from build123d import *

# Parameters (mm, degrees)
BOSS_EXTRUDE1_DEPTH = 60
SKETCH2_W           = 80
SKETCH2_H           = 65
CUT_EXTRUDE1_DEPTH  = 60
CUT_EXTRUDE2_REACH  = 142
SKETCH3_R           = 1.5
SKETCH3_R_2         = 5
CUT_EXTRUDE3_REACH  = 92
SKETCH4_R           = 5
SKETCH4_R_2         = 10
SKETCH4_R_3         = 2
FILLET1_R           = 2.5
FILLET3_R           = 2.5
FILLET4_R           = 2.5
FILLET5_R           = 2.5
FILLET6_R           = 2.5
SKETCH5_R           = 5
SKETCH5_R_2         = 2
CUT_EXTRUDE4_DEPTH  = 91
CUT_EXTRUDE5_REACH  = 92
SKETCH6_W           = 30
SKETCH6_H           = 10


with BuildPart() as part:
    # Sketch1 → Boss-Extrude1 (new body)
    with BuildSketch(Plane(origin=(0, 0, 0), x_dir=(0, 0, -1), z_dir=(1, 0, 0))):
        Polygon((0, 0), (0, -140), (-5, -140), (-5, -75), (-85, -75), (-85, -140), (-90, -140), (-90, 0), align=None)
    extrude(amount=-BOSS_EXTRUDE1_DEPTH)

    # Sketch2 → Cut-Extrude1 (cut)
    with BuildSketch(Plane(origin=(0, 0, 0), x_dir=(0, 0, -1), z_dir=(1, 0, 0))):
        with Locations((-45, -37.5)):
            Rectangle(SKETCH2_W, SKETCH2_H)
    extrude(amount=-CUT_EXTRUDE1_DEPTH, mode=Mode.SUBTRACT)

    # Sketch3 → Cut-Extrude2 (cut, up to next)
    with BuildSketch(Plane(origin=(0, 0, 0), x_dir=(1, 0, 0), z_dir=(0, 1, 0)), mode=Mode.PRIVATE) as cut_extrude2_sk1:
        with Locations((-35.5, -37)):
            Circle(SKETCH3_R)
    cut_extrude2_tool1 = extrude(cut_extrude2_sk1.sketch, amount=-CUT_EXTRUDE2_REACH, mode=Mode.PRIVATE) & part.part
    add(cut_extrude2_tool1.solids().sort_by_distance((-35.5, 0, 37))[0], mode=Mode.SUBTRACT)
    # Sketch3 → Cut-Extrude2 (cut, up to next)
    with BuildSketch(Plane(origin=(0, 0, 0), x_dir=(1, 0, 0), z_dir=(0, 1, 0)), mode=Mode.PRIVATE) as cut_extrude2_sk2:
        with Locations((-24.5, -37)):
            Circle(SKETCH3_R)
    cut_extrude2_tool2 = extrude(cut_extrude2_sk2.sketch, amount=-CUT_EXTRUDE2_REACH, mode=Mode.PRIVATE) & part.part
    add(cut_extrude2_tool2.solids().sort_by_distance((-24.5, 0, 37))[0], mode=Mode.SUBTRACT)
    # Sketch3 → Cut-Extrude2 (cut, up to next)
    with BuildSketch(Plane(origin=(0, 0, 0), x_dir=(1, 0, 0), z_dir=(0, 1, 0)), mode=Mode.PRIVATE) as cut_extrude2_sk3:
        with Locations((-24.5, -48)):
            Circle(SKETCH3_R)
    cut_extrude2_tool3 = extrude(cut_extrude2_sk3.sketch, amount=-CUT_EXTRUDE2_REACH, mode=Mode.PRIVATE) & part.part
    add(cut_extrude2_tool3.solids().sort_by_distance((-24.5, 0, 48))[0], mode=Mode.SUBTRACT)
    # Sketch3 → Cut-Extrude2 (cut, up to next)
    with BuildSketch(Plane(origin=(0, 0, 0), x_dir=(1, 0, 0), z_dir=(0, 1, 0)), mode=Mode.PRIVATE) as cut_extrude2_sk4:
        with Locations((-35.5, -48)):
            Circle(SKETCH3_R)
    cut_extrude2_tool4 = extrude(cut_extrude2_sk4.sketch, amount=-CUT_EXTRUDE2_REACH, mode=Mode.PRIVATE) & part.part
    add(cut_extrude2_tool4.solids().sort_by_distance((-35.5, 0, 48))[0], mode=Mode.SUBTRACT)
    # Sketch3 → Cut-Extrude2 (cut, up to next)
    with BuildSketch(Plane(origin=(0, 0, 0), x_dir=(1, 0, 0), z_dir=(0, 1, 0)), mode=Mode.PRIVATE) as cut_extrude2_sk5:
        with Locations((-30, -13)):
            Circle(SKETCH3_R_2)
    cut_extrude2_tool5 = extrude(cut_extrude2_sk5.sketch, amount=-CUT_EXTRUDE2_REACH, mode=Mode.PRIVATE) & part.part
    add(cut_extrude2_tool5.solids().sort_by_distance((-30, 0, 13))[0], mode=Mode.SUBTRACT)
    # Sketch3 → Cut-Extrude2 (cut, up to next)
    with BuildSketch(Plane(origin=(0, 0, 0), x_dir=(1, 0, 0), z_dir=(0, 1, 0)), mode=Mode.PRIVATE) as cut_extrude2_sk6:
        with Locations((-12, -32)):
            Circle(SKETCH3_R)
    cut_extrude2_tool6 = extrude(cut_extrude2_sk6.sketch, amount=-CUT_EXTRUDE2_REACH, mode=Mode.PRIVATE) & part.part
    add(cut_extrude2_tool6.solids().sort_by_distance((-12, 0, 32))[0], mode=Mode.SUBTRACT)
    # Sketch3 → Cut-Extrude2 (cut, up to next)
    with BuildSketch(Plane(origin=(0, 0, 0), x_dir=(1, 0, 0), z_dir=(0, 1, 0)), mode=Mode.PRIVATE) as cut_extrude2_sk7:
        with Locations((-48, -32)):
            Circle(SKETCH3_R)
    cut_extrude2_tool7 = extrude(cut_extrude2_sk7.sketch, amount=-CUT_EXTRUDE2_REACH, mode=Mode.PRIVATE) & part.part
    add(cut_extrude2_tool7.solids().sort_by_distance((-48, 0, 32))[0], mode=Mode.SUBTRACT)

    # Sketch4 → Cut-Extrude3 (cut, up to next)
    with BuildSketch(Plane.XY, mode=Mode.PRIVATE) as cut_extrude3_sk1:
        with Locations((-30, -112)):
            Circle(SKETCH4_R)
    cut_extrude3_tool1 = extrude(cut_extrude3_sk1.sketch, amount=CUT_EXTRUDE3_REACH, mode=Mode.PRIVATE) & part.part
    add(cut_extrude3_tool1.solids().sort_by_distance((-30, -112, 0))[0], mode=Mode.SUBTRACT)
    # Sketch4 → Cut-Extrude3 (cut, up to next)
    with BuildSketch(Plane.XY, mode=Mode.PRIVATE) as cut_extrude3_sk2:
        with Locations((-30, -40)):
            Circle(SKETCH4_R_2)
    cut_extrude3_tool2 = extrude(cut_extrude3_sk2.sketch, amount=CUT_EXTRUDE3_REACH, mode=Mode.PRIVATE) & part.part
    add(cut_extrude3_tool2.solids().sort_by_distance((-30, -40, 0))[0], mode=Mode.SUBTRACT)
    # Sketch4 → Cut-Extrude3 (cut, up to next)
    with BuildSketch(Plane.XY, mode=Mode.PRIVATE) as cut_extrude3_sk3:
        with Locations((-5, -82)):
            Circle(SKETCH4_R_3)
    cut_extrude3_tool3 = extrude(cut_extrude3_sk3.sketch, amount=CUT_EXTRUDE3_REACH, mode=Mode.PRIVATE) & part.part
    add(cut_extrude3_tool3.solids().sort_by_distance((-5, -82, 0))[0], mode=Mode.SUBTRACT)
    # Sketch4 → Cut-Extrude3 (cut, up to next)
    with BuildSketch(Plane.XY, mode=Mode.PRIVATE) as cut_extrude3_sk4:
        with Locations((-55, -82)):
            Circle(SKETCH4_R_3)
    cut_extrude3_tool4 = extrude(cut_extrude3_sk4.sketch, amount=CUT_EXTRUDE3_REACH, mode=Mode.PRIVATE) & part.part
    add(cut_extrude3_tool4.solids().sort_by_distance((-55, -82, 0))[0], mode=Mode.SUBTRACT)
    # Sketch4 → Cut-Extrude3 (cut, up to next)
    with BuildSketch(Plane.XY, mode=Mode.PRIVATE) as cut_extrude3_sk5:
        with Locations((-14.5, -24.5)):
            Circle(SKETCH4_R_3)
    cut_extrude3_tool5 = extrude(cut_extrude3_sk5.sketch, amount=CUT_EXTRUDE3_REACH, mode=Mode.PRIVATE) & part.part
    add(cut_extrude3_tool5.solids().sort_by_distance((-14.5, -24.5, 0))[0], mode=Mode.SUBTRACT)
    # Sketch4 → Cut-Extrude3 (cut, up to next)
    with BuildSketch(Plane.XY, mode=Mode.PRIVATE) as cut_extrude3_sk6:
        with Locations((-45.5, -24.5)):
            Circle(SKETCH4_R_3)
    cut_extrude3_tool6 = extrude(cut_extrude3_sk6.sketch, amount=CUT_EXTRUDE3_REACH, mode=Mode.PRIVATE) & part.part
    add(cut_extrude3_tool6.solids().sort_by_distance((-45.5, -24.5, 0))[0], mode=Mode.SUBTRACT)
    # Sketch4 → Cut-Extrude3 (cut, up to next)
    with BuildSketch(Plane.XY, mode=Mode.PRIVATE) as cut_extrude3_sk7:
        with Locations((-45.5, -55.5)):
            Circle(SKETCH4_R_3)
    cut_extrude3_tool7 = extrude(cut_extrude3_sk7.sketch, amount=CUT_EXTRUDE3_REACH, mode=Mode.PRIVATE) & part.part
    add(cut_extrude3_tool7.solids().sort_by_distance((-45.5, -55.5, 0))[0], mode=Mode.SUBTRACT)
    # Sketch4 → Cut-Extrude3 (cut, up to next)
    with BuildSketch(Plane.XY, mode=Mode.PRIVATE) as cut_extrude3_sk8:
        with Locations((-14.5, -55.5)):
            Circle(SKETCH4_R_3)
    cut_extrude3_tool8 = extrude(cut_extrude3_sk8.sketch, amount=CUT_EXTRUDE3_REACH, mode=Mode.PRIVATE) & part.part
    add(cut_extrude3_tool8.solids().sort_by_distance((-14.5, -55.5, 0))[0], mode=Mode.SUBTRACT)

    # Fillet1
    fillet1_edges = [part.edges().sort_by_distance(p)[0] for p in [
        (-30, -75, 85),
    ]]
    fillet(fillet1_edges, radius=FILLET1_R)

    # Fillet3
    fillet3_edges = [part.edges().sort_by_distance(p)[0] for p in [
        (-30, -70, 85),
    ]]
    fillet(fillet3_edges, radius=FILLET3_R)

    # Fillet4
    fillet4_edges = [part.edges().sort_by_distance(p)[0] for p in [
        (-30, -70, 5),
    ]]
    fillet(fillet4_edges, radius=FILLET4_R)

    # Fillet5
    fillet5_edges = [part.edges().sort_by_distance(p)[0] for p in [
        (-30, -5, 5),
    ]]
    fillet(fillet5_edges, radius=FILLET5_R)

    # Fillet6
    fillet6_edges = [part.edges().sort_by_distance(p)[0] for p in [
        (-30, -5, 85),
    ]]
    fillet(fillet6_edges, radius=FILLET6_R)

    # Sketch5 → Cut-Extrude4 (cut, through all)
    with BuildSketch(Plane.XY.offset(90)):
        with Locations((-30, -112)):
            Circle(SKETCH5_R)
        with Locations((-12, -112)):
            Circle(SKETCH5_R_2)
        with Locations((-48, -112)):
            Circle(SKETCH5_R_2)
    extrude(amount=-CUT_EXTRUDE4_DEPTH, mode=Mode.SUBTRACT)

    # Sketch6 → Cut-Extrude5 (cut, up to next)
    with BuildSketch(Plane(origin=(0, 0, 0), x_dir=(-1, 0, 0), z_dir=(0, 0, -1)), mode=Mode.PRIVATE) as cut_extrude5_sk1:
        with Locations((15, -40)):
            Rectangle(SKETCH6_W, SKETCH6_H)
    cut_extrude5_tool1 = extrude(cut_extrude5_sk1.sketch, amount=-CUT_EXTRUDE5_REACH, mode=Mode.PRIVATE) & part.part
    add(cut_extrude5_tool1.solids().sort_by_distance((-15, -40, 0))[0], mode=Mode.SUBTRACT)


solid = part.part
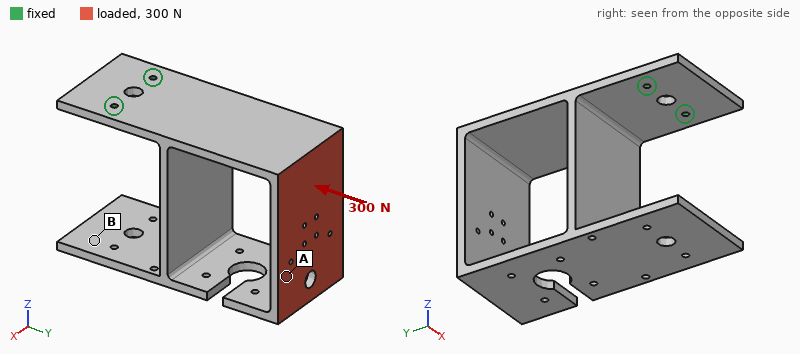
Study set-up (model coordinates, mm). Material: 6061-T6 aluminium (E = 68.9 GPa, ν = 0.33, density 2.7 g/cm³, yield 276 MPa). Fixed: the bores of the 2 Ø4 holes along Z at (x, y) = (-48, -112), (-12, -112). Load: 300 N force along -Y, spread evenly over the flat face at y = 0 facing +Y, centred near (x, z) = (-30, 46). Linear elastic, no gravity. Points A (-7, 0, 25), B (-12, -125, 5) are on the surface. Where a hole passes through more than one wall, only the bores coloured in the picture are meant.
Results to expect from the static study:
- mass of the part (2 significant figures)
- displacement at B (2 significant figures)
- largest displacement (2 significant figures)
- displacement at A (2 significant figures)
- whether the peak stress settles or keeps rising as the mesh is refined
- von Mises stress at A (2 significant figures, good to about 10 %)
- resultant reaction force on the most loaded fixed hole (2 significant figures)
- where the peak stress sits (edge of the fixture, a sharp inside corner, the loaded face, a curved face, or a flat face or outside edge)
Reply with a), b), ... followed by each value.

a) 350 g
b) 1.4 mm
c) 1.8 mm
d) 1.6 mm
e) keeps rising
f) 9.4 MPa
g) 150 N
h) edge of the fixture
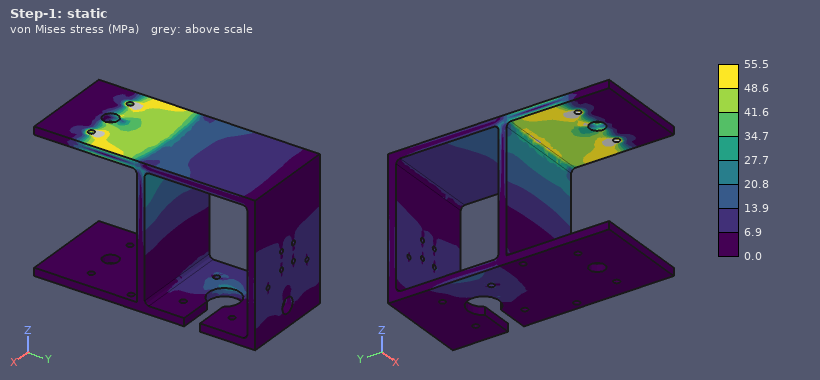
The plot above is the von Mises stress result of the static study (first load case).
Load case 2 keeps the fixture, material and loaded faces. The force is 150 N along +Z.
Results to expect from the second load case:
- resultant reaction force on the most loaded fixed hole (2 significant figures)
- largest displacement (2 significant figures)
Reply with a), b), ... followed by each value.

a) 76 N
b) 1.9 mm
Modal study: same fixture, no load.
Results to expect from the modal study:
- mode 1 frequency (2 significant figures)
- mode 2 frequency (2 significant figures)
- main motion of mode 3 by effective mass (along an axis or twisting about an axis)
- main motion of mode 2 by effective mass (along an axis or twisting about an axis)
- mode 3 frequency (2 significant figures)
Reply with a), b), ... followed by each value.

a) 110 Hz
b) 270 Hz
c) along Z
d) along X
e) 480 Hz
